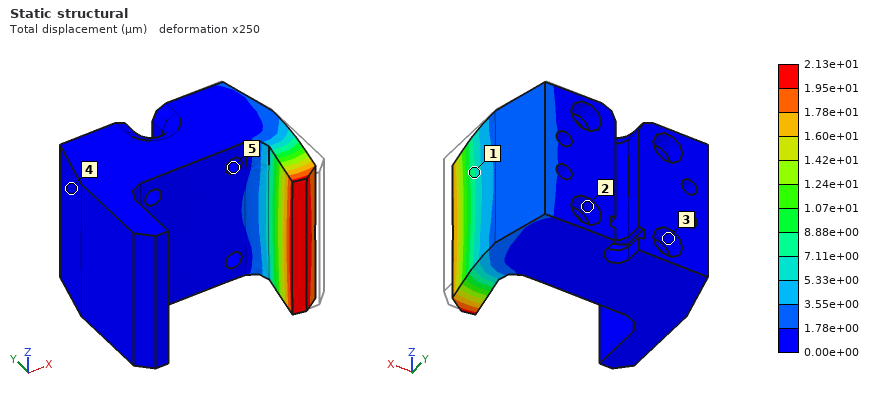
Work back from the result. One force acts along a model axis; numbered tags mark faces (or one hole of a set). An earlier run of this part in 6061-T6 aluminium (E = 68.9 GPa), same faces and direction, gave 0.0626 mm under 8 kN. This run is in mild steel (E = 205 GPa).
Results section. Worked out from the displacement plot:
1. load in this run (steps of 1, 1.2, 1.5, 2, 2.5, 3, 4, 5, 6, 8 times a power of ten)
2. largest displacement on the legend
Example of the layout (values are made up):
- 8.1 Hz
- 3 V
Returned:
- 8 kN
- 2.13e+01 µm
